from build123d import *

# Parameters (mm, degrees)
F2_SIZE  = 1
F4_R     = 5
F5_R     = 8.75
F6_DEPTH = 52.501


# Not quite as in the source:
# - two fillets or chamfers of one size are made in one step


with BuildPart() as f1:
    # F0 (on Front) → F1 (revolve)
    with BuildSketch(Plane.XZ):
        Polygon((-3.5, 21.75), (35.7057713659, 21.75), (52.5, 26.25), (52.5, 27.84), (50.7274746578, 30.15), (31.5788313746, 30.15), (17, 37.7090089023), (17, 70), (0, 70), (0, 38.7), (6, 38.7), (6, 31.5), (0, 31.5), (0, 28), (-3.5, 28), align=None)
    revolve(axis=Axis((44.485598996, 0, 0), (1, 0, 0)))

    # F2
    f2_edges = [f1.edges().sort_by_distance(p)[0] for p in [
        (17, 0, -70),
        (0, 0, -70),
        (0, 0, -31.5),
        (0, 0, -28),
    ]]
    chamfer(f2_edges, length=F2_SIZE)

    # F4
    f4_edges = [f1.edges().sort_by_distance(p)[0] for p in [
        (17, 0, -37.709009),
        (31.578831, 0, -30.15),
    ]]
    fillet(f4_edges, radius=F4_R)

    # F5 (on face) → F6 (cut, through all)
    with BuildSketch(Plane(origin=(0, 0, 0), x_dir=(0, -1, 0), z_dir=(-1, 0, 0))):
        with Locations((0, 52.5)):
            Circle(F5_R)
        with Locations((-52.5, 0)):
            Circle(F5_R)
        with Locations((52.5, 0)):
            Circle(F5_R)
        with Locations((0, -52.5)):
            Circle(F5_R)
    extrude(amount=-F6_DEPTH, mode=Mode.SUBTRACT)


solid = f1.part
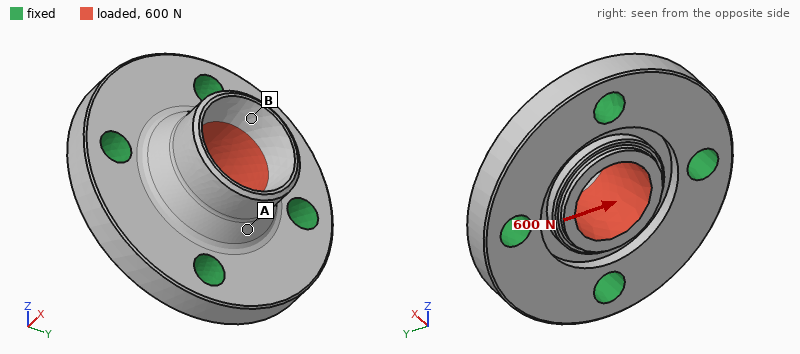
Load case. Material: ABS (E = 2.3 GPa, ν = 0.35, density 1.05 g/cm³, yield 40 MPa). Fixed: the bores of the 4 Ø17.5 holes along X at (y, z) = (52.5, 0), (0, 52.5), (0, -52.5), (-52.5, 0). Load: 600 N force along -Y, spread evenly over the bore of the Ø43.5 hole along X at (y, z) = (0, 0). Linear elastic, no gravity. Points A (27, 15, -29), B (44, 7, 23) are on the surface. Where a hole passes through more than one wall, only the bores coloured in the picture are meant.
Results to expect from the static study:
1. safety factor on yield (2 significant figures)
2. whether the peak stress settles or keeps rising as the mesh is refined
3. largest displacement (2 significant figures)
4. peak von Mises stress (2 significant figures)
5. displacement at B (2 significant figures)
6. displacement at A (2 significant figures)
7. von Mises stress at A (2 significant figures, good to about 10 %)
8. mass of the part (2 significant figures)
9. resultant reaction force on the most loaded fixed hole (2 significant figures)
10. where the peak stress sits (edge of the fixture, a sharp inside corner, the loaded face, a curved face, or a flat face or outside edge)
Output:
44
settles
6.3 µm
0.91 MPa
5.7 µm
4.8 µm
0.17 MPa
280 g
190 N
a curved face
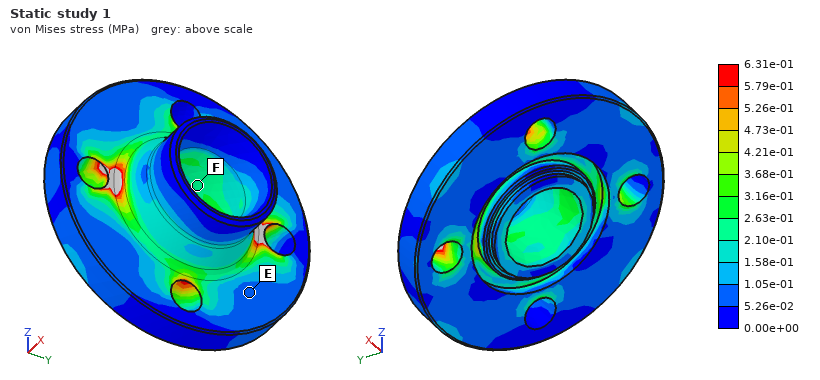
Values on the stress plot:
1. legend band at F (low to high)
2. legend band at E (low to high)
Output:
2.10e-01 to 2.63e-01 MPa
5.26e-02 to 1.05e-01 MPa
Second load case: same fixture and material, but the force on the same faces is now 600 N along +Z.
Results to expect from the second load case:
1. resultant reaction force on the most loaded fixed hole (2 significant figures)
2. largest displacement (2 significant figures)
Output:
190 N
6.3 µm
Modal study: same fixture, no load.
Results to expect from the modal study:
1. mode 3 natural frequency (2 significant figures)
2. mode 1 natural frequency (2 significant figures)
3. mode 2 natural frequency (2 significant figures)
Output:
3300 Hz
3200 Hz
3300 Hz
